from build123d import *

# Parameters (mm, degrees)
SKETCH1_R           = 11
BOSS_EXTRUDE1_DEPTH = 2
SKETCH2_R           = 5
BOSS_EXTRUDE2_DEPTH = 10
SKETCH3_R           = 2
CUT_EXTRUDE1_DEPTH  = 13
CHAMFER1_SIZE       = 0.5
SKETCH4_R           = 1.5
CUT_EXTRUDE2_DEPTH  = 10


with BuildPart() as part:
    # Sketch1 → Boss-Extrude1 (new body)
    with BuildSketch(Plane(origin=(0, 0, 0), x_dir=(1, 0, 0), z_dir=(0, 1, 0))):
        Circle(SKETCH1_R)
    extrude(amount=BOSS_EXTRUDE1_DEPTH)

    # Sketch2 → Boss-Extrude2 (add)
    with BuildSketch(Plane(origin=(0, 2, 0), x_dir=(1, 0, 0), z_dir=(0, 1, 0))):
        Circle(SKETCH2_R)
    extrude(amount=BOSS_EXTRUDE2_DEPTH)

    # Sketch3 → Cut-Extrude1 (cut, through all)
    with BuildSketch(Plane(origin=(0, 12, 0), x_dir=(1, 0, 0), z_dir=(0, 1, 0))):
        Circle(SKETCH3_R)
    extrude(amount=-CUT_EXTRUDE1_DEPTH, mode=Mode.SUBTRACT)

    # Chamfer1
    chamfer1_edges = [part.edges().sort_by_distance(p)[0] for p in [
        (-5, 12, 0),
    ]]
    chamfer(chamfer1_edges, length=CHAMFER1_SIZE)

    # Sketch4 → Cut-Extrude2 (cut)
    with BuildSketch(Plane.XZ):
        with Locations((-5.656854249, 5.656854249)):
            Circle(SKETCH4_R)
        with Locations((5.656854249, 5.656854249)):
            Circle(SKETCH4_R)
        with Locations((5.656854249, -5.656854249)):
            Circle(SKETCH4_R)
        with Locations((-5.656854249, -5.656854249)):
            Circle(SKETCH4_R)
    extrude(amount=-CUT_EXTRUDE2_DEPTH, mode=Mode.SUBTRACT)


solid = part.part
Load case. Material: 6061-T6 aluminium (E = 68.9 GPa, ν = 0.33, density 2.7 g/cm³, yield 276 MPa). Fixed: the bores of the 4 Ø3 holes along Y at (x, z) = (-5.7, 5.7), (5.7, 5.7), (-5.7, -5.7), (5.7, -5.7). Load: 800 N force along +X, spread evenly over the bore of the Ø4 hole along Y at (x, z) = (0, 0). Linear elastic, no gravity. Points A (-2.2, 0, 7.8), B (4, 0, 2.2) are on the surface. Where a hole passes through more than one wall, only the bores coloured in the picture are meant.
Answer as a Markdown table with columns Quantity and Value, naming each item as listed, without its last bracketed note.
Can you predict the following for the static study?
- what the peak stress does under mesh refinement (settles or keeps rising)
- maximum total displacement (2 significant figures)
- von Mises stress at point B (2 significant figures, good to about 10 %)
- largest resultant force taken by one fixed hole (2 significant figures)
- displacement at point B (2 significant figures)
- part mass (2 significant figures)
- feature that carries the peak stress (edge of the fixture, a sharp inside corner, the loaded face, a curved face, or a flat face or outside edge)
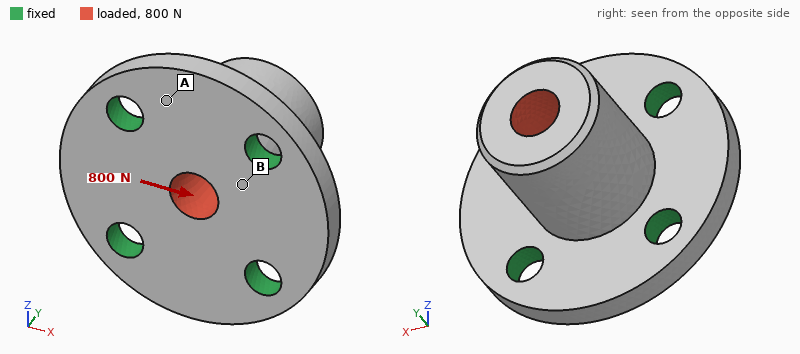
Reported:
| Quantity | Value |
|---|---|
| what the peak stress does under mesh refinement | keeps rising |
| maximum total displacement | 16 µm |
| von Mises stress at point B | 24 MPa |
| largest resultant force taken by one fixed hole | 300 N |
| displacement at point B | 3.0 µm |
| part mass | 3.6 g |
| feature that carries the peak stress | edge of the fixture |
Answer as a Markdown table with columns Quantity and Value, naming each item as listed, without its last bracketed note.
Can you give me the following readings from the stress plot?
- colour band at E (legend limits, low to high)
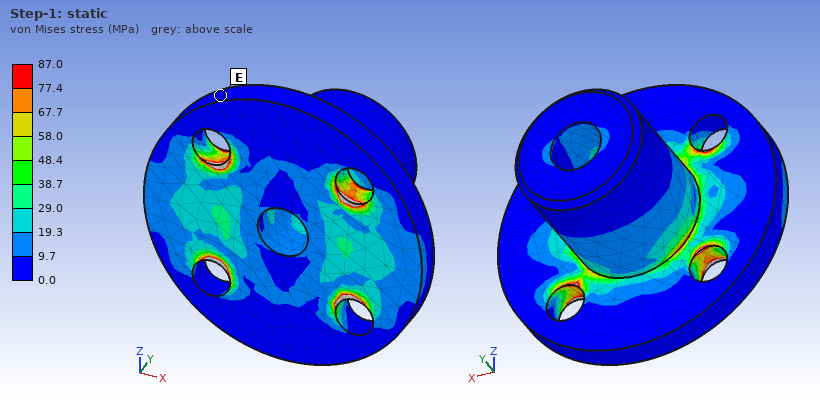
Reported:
| Quantity | Value |
|---|---|
| colour band at E | 0.0 to 9.7 MPa |
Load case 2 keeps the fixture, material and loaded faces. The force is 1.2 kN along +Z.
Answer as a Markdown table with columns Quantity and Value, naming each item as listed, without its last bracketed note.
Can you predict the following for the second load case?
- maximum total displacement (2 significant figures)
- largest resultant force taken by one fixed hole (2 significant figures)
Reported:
| Quantity | Value |
|---|---|
| maximum total displacement | 24 µm |
| largest resultant force taken by one fixed hole | 450 N |
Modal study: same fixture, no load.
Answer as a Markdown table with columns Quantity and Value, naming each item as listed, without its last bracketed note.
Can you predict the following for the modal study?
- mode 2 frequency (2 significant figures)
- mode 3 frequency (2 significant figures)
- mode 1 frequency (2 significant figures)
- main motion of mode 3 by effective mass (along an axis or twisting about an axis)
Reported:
| Quantity | Value |
|---|---|
| mode 2 frequency | 29 kHz |
| mode 3 frequency | 48 kHz |
| mode 1 frequency | 29 kHz |
| main motion of mode 3 by effective mass | along Y |
